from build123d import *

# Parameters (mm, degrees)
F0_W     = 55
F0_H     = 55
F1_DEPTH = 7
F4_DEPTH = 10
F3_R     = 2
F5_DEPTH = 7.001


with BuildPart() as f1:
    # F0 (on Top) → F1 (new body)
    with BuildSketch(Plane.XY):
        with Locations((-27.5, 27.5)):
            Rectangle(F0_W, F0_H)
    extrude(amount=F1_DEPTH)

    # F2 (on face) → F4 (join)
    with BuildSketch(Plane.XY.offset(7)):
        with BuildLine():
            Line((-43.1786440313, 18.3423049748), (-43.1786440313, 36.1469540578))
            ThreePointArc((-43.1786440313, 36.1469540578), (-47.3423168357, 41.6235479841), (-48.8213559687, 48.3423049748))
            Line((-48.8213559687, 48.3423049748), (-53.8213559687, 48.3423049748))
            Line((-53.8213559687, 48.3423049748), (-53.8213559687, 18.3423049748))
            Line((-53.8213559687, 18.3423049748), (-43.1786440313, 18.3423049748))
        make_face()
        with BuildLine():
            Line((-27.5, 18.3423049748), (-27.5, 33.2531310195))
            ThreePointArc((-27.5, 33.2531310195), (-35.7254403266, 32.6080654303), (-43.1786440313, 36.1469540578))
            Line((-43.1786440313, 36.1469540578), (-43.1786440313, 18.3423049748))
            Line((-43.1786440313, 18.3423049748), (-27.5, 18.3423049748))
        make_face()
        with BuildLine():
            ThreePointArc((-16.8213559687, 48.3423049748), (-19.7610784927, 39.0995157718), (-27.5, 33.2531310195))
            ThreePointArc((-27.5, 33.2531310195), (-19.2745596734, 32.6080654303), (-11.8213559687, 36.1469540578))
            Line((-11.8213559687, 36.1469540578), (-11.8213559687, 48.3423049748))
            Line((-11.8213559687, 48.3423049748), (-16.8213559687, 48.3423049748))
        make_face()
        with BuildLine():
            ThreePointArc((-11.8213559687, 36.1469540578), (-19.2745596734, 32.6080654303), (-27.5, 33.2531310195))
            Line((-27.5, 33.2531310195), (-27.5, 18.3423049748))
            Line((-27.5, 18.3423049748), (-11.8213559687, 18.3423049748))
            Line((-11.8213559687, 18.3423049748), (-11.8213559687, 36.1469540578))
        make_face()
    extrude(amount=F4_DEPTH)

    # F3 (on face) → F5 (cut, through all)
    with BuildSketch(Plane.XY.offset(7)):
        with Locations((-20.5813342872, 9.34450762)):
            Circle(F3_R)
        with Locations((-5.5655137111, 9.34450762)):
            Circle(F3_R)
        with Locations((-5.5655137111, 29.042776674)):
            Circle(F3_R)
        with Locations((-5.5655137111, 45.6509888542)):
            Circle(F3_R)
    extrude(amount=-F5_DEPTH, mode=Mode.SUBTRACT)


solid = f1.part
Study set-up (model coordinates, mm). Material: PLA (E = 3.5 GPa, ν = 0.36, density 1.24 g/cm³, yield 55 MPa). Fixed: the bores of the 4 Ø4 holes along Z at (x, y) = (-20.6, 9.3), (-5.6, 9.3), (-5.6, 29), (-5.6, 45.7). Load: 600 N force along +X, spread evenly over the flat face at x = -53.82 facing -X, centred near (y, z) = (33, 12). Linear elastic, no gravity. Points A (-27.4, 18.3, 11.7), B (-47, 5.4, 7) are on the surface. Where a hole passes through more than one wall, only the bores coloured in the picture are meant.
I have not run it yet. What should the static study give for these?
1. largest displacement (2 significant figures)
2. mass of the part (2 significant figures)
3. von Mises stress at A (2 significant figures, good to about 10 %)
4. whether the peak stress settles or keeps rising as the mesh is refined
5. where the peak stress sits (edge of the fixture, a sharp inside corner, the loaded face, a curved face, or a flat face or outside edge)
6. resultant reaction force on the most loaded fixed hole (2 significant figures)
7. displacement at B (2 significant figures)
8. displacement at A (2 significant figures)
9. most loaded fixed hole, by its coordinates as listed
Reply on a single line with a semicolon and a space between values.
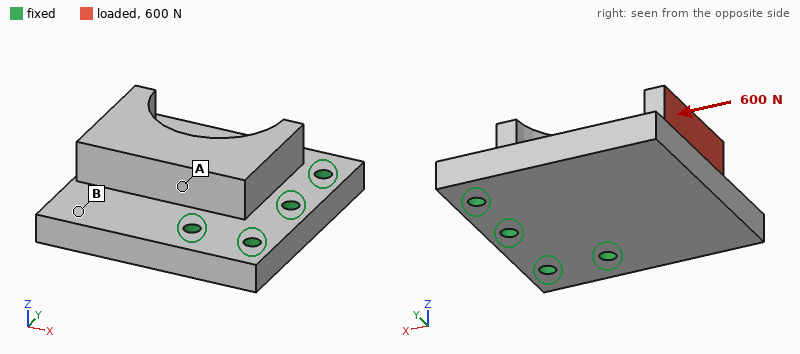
0.37 mm; 36 g; 3.2 MPa; keeps rising; edge of the fixture; 300 N; 0.14 mm; 0.082 mm; (-5.6, 29)
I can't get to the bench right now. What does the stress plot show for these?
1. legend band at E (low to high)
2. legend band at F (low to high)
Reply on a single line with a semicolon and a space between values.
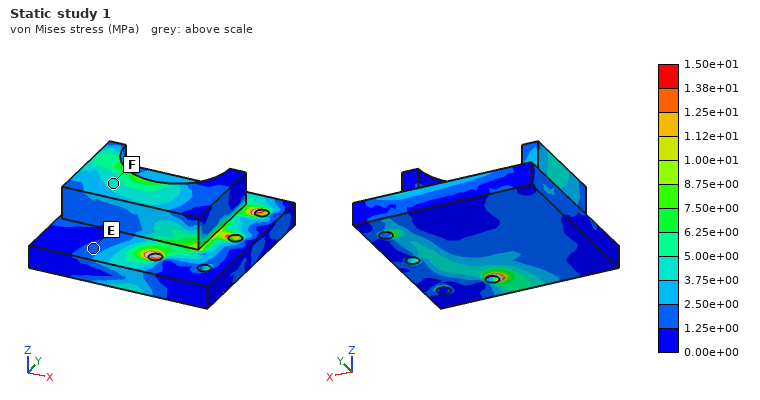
1.25e+00 to 2.50e+00 MPa; 3.75e+00 to 5.00e+00 MPa
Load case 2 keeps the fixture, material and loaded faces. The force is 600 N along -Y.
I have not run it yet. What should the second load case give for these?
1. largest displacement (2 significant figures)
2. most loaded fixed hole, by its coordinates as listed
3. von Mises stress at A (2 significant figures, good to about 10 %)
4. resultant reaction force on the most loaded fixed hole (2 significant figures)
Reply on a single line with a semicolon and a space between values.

0.29 mm; (-20.6, 9.3); 4.4 MPa; 650 N
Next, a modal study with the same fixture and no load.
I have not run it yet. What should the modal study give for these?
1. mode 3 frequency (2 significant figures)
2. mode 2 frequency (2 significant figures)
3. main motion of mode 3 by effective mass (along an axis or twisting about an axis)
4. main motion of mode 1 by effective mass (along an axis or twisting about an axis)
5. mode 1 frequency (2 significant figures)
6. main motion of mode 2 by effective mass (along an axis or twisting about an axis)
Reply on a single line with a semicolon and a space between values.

3700 Hz; 2800 Hz; along Y; along Z; 1000 Hz; twisting about X
